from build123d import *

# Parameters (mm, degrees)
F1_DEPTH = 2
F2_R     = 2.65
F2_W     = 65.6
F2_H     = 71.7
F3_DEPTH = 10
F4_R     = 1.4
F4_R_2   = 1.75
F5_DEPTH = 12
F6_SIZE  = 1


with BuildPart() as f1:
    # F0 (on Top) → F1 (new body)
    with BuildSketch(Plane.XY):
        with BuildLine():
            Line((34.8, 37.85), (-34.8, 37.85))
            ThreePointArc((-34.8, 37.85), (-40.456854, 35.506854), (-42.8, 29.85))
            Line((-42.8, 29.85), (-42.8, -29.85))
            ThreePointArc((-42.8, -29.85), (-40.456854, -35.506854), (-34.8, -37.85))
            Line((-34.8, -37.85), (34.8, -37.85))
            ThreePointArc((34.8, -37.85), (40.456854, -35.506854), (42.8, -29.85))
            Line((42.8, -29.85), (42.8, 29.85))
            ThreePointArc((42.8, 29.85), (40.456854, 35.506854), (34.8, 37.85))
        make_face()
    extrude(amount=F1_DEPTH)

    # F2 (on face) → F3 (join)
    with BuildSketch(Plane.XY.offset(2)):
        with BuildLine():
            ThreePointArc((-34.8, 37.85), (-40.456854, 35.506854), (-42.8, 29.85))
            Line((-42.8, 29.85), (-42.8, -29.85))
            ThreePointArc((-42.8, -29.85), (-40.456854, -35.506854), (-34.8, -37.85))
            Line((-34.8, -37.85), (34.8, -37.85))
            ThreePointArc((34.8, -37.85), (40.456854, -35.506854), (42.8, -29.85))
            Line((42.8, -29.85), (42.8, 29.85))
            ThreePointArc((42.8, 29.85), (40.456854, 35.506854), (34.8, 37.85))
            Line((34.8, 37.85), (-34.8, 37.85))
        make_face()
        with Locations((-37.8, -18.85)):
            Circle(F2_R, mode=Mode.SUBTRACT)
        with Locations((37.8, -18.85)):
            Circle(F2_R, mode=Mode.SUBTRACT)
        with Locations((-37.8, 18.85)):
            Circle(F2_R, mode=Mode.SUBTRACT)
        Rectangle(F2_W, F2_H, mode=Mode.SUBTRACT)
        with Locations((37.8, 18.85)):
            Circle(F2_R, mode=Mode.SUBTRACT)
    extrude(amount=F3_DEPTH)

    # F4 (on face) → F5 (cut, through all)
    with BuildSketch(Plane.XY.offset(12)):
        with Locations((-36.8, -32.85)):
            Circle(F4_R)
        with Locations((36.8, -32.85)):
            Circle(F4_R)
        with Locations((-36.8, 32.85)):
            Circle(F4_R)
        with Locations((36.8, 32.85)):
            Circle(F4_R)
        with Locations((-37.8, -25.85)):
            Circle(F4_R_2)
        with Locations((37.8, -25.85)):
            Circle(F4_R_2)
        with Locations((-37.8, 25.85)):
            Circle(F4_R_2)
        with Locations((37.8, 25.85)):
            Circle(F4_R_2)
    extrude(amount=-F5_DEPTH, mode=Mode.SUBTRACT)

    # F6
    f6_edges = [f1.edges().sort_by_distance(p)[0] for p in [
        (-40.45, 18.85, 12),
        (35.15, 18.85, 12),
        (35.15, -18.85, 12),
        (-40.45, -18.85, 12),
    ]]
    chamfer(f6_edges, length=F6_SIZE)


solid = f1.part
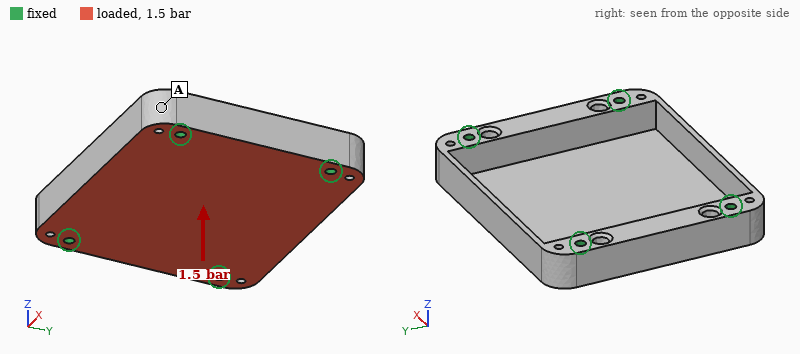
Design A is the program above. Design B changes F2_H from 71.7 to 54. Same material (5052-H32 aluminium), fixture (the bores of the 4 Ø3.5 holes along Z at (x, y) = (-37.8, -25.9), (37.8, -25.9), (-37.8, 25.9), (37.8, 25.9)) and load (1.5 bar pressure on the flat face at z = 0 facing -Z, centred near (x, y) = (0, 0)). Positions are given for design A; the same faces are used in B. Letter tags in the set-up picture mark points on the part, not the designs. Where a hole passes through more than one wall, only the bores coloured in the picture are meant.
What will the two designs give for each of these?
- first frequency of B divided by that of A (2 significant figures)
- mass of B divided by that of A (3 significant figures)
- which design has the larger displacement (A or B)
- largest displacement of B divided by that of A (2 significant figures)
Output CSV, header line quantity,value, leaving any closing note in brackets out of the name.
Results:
quantity,value
first frequency of B divided by that of A,1.5
mass of B divided by that of A,1.41
which design has the larger displacement,A
largest displacement of B divided by that of A,0.46
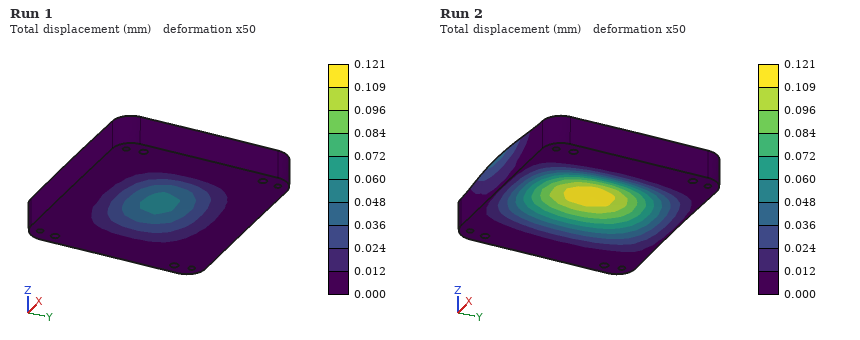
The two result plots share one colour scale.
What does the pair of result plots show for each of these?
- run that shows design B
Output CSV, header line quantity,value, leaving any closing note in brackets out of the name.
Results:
quantity,value
run that shows design B,Run 1
